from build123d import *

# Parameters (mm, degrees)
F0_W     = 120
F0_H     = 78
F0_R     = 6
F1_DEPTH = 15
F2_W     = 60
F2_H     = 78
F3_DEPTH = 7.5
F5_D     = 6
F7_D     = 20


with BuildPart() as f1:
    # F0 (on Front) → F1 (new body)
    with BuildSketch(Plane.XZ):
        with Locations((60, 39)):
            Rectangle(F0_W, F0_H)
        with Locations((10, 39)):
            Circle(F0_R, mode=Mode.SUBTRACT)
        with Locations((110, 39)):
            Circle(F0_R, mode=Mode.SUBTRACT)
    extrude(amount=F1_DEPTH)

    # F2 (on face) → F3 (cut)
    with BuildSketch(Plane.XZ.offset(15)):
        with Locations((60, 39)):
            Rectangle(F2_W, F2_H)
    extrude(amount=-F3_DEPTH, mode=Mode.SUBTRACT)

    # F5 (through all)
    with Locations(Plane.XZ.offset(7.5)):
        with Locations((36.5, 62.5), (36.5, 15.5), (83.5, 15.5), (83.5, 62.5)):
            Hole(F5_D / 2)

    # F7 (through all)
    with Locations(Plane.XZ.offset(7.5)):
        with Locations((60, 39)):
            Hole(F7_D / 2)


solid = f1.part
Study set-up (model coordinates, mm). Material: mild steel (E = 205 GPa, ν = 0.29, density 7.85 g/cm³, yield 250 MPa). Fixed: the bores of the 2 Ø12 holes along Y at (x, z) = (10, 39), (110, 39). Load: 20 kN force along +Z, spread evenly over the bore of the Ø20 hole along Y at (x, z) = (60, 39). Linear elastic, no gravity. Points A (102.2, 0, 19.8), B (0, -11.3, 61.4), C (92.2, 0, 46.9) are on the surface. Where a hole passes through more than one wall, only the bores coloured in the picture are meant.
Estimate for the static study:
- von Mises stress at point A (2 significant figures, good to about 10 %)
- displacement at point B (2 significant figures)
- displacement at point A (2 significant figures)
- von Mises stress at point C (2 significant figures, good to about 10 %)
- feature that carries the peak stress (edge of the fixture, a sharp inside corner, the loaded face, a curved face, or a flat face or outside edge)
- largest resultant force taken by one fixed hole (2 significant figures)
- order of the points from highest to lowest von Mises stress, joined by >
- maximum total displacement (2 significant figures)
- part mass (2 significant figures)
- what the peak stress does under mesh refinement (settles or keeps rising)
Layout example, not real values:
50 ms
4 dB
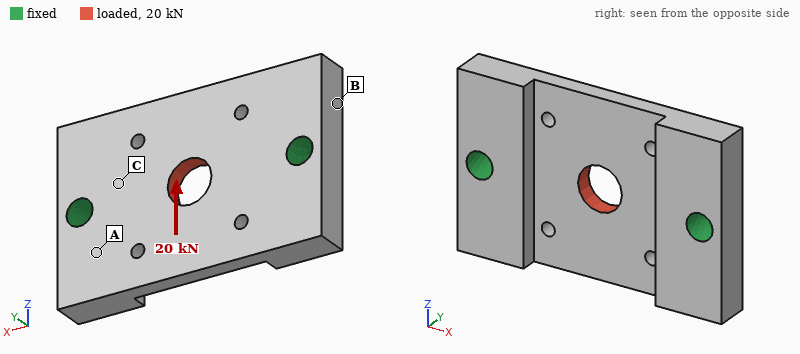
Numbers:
24 MPa
4.2 µm
4.7 µm
42 MPa
edge of the fixture
10 kN
C > A > B
18 µm
770 g
keeps rising
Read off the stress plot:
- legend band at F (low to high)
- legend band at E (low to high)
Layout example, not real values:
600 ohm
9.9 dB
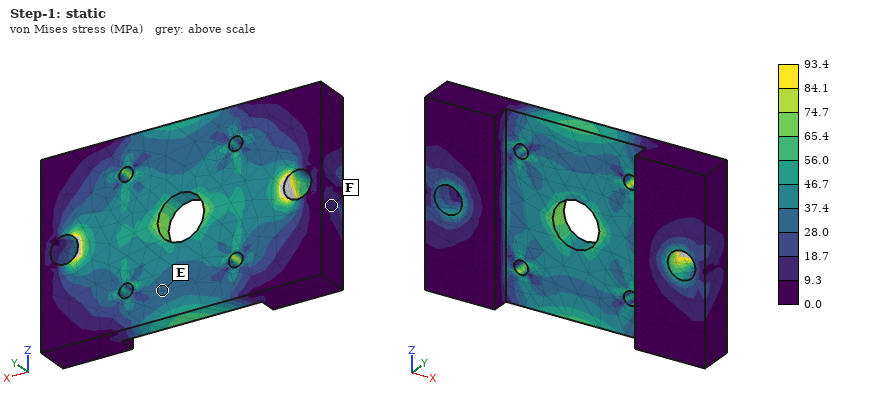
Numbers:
9.3 to 18.7 MPa
28.0 to 37.4 MPa
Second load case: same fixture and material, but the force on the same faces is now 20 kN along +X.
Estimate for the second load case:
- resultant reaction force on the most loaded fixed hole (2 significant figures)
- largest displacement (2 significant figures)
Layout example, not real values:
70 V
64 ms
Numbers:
10 kN
8.2 µm
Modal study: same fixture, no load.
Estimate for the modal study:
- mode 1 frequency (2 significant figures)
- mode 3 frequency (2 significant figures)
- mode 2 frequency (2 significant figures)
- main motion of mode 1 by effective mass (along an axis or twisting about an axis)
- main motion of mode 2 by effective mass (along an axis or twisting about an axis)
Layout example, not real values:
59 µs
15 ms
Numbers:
5200 Hz
7600 Hz
5500 Hz
twisting about X
along Y
